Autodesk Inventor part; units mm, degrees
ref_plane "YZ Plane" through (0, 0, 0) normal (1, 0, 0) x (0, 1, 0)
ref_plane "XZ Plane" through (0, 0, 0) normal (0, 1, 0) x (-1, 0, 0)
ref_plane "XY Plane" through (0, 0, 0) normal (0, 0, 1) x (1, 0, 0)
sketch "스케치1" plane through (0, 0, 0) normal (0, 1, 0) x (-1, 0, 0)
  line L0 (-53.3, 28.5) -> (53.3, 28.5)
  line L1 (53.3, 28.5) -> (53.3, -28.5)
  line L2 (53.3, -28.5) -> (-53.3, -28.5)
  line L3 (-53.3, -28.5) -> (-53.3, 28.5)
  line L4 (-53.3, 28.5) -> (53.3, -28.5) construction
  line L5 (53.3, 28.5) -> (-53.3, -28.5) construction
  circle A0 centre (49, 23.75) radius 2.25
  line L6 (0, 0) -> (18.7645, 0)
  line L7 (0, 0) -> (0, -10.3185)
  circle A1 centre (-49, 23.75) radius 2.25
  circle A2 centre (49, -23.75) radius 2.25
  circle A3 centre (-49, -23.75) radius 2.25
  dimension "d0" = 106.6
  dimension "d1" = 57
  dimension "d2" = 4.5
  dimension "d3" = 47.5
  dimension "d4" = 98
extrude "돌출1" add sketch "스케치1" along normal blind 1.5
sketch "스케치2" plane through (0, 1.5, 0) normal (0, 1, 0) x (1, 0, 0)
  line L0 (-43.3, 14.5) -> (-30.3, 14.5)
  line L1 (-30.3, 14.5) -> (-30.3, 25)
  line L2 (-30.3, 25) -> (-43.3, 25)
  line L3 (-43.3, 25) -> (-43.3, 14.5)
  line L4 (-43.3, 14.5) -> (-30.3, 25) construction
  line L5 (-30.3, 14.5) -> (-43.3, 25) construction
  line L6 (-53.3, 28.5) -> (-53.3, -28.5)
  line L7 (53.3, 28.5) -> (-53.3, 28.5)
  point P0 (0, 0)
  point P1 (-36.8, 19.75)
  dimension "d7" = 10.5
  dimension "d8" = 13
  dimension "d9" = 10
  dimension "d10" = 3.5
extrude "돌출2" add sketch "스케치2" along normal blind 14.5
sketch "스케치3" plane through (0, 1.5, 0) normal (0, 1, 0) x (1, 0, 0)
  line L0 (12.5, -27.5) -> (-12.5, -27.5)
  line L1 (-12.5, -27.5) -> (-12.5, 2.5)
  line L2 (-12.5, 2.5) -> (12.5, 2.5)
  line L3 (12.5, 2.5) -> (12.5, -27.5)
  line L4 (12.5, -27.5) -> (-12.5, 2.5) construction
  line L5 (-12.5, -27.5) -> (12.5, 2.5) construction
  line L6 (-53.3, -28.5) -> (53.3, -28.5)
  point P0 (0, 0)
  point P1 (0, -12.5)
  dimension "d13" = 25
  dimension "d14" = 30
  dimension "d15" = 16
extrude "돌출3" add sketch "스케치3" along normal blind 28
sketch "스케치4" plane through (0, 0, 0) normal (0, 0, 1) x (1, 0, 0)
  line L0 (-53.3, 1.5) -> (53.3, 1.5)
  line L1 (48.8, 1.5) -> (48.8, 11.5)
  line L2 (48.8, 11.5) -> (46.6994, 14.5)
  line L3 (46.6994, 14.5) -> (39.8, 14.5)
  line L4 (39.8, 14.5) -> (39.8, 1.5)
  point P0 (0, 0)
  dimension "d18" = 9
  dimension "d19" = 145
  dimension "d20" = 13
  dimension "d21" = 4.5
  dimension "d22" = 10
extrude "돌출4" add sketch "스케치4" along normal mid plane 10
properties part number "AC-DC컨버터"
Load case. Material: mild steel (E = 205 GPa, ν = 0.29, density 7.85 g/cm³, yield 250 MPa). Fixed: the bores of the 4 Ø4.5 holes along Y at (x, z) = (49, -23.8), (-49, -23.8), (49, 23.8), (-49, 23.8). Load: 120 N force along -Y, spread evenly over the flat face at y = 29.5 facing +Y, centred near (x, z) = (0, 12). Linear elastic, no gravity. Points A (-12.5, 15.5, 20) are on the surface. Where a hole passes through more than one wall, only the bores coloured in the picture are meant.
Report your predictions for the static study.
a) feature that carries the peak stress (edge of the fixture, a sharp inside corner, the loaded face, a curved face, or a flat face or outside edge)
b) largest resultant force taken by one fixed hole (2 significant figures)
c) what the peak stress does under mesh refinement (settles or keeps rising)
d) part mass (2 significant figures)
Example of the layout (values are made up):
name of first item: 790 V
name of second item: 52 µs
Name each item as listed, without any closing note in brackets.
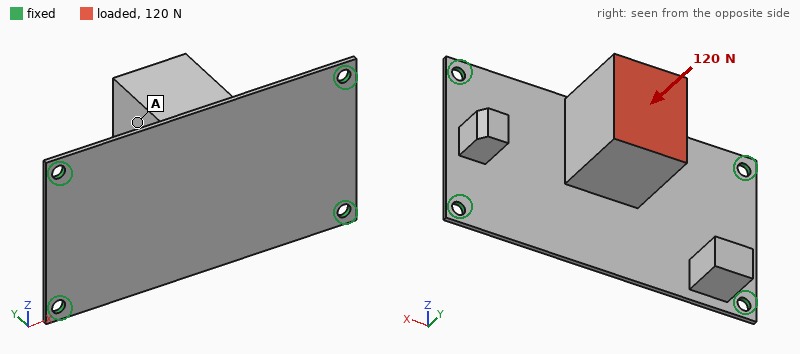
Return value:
feature that carries the peak stress: edge of the fixture
largest resultant force taken by one fixed hole: 53 N
what the peak stress does under mesh refinement: keeps rising
part mass: 260 g
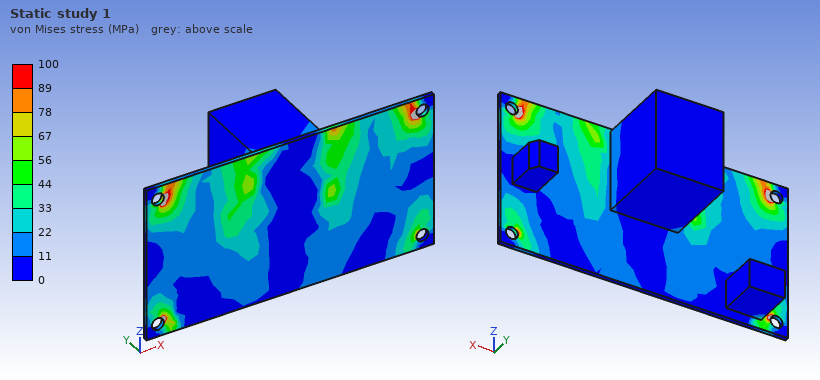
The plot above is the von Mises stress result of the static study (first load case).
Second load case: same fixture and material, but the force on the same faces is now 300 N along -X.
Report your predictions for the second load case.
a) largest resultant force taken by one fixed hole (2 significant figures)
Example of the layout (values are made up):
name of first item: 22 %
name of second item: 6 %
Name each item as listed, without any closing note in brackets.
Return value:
largest resultant force taken by one fixed hole: 120 N
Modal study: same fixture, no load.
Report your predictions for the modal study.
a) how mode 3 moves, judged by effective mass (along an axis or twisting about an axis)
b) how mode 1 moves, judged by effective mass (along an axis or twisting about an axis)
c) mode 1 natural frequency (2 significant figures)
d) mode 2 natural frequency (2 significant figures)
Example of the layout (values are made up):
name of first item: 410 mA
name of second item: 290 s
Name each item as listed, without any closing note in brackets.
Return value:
how mode 3 moves, judged by effective mass: along X
how mode 1 moves, judged by effective mass: along Y
mode 1 natural frequency: 380 Hz
mode 2 natural frequency: 520 Hz
